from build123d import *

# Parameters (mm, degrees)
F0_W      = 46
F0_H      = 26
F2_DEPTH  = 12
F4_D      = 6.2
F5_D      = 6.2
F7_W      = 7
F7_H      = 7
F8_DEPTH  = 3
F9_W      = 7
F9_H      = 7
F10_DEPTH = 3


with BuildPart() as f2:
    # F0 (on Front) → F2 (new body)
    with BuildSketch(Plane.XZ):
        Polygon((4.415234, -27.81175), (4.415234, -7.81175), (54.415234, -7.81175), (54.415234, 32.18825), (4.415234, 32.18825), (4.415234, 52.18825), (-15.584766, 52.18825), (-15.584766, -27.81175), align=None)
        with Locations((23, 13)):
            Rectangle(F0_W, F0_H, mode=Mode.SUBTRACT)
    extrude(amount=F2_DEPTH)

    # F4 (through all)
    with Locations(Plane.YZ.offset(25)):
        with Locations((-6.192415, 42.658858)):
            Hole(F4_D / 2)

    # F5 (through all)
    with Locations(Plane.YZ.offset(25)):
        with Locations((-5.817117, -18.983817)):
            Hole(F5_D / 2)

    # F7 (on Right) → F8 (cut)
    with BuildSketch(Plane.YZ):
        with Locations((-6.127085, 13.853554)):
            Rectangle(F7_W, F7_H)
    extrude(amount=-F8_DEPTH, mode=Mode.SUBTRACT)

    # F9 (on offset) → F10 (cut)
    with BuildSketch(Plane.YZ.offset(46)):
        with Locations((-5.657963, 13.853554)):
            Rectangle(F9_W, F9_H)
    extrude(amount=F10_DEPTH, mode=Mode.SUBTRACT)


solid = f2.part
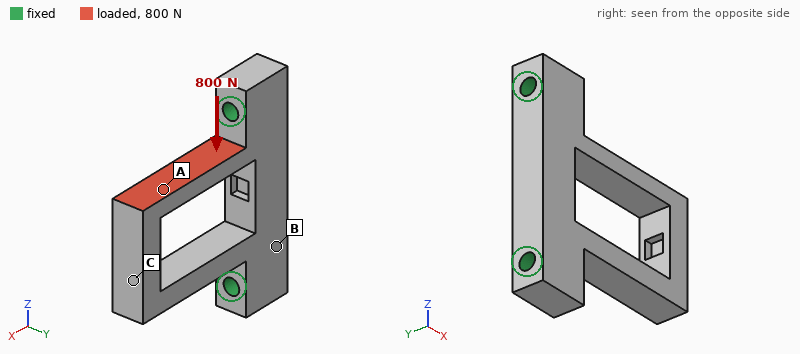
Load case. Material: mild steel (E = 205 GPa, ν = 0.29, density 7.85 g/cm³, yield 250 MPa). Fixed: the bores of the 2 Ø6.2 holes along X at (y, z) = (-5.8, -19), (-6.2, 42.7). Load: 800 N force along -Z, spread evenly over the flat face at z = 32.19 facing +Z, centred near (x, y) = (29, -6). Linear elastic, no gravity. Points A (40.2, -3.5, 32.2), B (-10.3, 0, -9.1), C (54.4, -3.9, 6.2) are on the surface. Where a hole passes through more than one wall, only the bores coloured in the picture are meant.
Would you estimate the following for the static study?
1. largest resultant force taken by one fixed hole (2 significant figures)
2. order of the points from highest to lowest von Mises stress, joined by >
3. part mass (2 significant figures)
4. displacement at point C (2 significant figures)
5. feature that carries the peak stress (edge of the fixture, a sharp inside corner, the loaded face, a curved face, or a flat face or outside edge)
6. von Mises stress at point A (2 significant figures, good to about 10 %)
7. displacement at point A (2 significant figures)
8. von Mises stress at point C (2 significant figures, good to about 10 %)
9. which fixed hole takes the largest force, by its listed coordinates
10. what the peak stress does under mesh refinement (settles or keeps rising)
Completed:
660 N
A > C > B
210 g
38 µm
a sharp inside corner
35 MPa
37 µm
23 MPa
(-6.2, 42.7)
keeps rising
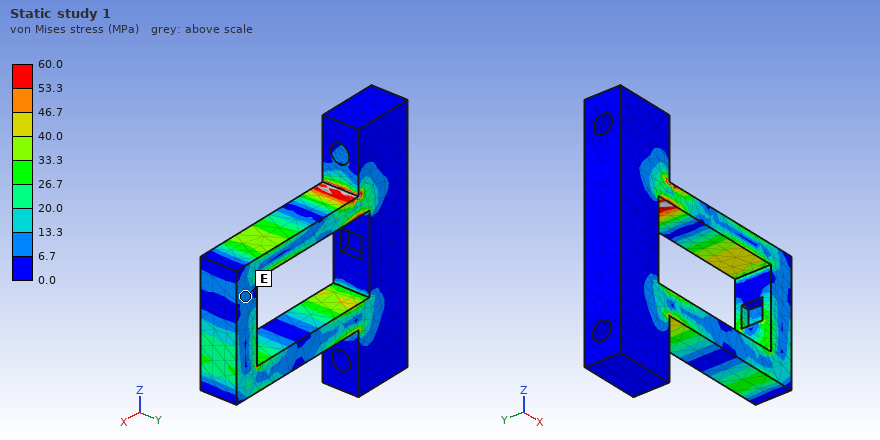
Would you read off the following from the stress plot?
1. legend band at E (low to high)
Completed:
6.7 to 13.3 MPa
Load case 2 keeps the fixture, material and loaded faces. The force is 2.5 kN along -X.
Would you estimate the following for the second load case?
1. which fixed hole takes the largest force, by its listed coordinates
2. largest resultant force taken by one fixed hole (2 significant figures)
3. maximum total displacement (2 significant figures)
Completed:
(-6.2, 42.7)
2.4 kN
19 µm
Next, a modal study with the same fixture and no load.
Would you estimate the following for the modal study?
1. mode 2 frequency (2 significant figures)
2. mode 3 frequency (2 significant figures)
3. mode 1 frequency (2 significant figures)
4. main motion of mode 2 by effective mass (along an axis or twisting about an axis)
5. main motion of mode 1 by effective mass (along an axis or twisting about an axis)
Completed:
2500 Hz
4400 Hz
2000 Hz
along Z
along Y
